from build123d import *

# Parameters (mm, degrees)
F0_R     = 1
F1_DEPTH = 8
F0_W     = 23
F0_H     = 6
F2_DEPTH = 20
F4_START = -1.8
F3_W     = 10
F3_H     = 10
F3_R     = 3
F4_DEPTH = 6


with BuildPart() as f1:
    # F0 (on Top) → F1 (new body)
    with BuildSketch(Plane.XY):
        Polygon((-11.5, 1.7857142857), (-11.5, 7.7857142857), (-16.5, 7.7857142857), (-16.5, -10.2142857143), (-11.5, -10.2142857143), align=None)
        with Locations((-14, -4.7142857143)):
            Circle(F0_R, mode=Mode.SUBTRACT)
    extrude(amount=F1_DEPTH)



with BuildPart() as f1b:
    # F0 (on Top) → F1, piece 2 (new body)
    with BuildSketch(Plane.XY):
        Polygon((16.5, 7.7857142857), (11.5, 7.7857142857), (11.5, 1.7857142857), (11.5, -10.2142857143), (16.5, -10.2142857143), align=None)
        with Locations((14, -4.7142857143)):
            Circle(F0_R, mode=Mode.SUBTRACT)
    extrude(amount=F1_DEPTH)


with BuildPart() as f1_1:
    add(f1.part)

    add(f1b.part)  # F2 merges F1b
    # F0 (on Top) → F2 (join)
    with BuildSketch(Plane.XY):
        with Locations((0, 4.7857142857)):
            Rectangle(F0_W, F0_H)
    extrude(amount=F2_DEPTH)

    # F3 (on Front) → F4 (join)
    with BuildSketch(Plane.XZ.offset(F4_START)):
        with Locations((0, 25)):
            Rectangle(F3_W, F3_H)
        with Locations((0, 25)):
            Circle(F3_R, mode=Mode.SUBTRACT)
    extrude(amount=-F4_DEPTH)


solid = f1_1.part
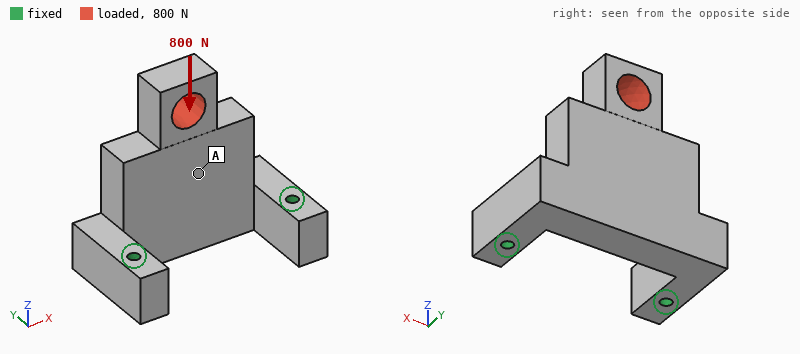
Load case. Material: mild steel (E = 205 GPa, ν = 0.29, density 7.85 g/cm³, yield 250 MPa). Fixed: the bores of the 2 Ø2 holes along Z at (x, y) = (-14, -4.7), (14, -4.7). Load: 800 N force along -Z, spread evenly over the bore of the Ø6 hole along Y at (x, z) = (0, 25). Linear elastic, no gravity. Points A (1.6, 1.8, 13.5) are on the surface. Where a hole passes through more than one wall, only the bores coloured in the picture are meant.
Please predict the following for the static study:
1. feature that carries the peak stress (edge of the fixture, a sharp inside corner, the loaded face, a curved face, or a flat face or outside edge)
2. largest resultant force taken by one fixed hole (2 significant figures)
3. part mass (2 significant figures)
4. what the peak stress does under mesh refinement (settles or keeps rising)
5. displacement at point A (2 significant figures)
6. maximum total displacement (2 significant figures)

edge of the fixture
400 N
36 g
keeps rising
5.6 µm
14 µm
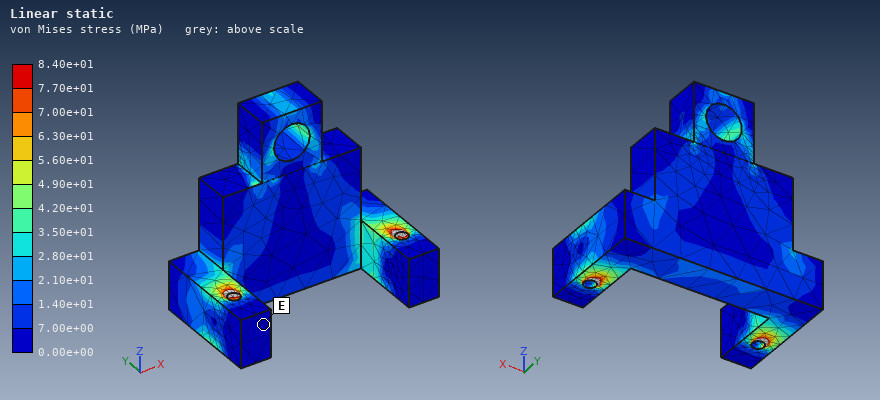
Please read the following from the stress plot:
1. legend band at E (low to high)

0.00e+00 to 7.00e+00 MPa
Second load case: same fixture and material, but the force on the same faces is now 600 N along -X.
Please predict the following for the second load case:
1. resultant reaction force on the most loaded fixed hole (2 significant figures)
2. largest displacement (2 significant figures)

540 N
17 µm
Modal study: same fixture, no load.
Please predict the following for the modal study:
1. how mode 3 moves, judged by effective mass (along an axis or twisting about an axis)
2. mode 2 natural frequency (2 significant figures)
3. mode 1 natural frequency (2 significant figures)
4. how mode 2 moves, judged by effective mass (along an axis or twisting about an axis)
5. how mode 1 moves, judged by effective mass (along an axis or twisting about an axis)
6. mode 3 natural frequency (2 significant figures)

along Z
12 kHz
5900 Hz
along X
along Y
15 kHz
